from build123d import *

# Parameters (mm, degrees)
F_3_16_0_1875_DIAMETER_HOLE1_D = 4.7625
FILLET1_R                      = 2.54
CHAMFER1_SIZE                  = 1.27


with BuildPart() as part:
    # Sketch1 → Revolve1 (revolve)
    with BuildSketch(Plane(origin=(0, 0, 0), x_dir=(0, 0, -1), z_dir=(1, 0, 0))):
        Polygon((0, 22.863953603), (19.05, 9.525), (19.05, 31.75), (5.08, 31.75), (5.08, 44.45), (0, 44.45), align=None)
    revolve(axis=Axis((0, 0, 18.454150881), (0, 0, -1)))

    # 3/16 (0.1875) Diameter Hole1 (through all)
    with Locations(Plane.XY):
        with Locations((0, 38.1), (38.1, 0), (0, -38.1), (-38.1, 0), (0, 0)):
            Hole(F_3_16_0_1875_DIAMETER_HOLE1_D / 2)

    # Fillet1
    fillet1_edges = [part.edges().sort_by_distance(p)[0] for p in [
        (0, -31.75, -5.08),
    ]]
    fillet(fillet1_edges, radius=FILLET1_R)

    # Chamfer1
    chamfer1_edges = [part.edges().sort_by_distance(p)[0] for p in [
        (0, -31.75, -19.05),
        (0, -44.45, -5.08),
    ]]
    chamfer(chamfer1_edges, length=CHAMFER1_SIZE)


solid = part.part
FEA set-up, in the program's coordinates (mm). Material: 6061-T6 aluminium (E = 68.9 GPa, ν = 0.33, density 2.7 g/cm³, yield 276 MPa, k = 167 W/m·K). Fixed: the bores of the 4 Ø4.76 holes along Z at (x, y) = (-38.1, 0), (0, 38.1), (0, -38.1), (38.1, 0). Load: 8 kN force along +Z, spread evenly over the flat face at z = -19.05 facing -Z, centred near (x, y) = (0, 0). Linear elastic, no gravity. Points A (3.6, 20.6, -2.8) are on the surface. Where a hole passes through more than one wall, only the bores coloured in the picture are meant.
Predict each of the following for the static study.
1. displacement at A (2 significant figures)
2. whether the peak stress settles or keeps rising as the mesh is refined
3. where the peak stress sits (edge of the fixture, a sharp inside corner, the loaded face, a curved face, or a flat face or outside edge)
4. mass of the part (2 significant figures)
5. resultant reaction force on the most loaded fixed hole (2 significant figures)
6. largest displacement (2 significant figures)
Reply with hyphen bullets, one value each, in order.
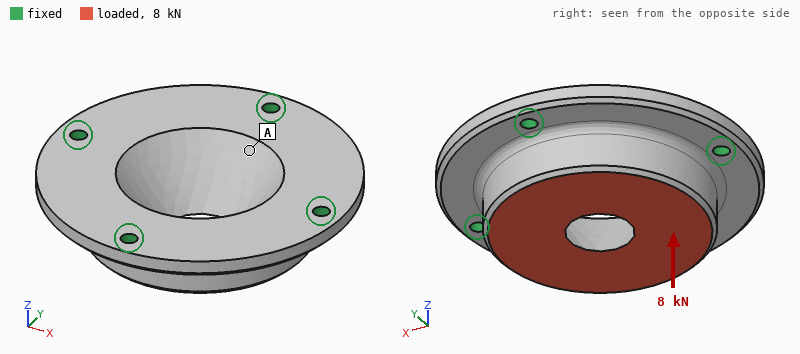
- 18 µm
- keeps rising
- edge of the fixture
- 160 g
- 2.5 kN
- 23 µm
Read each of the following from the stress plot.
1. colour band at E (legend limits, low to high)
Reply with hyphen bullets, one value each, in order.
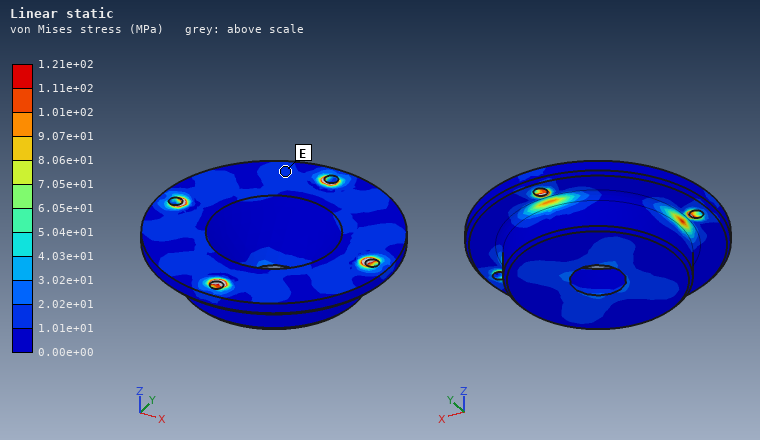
- 1.01e+01 to 2.02e+01 MPa
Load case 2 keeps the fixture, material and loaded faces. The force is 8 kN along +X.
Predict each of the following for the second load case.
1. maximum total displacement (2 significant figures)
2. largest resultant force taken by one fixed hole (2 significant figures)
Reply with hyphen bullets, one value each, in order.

- 16 µm
- 3.0 kN
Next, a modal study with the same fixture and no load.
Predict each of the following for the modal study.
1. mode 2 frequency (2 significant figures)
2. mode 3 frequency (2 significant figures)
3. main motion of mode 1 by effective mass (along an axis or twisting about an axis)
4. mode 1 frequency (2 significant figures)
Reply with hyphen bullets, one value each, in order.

- 10 kHz
- 10 kHz
- along Z
- 9300 Hz
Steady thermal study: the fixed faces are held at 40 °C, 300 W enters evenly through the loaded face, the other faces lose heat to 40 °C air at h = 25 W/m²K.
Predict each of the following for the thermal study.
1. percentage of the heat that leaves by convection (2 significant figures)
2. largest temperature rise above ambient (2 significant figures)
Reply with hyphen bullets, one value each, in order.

- 3.6 %
- 52 K
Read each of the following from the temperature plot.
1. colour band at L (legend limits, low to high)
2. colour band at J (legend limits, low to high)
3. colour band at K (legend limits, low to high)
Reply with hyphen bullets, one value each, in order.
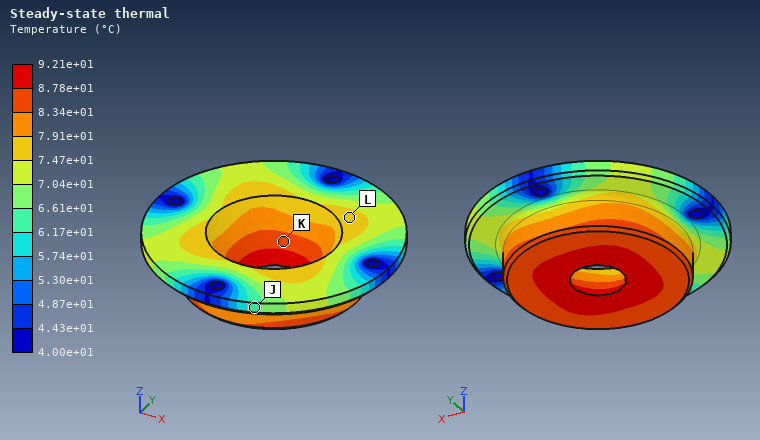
- 7.47e+01 to 7.91e+01 °C
- 6.17e+01 to 6.61e+01 °C
- 8.34e+01 to 8.78e+01 °C
